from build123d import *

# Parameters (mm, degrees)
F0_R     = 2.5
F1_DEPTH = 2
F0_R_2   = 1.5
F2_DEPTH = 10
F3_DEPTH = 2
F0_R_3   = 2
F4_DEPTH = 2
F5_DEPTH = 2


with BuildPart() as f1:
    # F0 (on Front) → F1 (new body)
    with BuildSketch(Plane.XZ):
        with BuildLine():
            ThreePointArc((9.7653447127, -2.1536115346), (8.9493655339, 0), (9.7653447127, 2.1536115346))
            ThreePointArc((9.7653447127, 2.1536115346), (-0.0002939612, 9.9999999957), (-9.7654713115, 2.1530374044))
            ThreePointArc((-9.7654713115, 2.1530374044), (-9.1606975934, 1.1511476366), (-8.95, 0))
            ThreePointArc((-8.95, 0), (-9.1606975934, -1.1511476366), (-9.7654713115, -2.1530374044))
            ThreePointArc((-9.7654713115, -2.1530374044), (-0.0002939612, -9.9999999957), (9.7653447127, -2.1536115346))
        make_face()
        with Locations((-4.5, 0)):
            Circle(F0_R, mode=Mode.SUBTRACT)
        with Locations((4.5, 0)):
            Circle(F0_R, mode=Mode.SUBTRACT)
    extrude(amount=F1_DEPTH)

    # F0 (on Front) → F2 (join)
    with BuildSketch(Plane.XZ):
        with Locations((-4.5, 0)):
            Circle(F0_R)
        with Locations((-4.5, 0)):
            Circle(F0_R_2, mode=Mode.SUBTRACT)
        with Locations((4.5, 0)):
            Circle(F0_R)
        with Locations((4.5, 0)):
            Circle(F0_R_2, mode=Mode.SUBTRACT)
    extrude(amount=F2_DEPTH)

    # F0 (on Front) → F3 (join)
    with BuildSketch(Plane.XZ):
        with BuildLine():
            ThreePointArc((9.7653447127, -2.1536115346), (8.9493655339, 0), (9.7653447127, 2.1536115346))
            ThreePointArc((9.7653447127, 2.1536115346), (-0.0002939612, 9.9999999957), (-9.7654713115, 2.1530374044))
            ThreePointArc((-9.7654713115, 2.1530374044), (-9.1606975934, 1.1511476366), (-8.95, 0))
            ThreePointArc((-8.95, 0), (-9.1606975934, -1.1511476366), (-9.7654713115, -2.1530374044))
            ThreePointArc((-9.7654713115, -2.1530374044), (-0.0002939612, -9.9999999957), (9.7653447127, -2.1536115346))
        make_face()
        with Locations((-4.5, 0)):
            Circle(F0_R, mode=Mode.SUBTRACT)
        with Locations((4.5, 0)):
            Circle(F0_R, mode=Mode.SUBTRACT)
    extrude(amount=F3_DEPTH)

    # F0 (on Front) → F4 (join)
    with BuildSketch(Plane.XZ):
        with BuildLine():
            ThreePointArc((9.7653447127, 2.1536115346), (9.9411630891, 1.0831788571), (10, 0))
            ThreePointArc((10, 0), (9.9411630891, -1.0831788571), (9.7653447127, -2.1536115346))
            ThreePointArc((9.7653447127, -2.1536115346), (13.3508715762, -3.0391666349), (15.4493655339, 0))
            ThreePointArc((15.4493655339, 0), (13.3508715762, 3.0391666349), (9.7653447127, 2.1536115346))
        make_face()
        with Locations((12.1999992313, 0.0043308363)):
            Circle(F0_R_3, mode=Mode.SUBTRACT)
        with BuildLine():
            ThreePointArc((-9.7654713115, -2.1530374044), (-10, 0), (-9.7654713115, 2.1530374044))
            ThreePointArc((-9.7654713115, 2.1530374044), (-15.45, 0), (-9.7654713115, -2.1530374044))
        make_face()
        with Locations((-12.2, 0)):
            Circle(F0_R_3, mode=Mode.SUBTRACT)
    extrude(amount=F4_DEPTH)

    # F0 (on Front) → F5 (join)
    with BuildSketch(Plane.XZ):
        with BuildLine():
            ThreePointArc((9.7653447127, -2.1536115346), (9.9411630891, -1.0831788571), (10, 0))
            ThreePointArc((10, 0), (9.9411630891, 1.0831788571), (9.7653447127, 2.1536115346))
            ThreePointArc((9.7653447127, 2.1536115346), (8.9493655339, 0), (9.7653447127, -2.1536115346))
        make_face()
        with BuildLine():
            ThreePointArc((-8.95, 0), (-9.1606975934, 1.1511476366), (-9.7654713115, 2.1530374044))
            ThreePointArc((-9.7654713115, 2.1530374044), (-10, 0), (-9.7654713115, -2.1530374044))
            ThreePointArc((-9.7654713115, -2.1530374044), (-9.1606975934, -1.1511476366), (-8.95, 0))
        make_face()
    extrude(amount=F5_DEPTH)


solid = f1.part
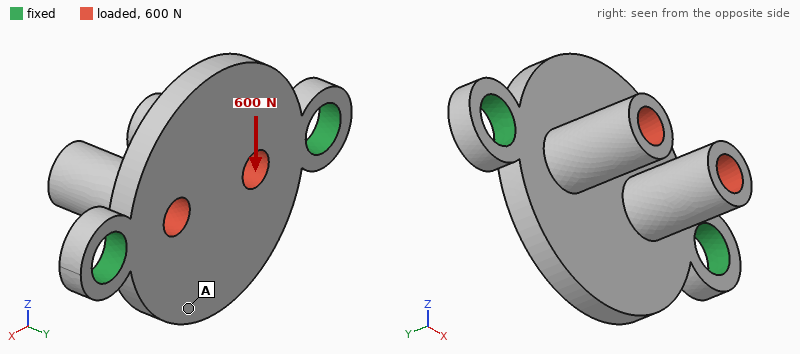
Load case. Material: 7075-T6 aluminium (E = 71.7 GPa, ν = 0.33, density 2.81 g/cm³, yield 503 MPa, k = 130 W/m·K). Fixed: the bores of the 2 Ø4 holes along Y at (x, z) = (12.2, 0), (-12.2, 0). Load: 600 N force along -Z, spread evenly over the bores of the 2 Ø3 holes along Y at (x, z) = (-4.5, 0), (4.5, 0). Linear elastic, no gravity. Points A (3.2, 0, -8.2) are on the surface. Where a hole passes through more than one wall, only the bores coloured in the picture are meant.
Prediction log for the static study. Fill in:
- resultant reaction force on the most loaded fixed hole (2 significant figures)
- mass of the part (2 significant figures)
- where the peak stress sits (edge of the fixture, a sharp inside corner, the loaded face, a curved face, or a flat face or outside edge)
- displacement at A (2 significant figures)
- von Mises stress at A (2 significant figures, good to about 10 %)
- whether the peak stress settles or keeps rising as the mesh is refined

300 N
2.4 g
a sharp inside corner
0.090 mm
40 MPa
keeps rising
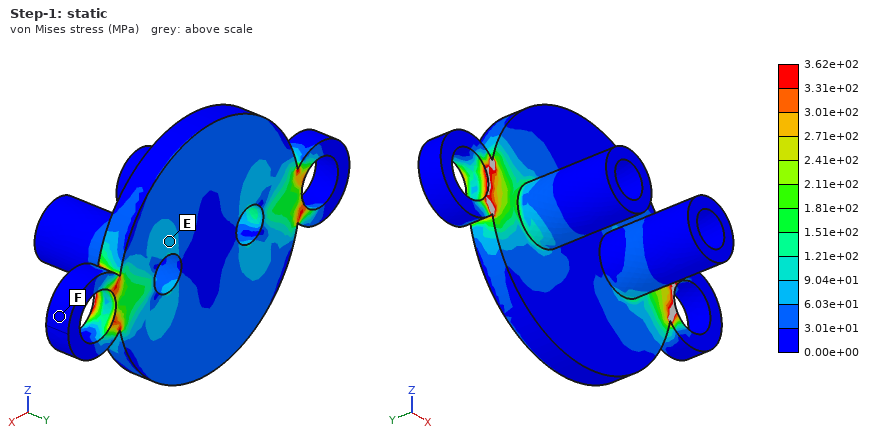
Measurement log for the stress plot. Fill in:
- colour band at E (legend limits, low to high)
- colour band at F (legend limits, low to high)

6.03e+01 to 9.04e+01 MPa
0.00e+00 to 3.01e+01 MPa
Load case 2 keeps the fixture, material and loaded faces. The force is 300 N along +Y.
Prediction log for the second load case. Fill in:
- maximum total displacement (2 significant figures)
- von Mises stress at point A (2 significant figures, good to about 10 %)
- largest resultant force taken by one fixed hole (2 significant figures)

31 µm
24 MPa
150 N
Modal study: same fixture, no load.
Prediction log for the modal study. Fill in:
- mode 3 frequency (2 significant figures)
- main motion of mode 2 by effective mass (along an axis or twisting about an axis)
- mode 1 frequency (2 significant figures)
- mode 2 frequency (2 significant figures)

24 kHz
along Y
9100 Hz
12 kHz
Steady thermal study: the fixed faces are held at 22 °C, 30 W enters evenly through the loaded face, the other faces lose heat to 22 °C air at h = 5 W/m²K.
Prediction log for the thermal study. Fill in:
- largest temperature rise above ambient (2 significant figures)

77 K
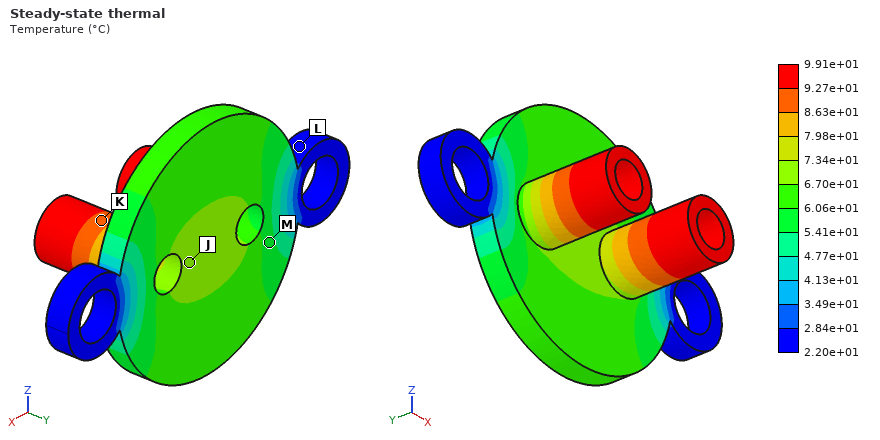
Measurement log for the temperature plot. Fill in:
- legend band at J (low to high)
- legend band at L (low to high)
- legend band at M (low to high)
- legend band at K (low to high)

6.70e+01 to 7.34e+01 °C
2.20e+01 to 2.84e+01 °C
5.41e+01 to 6.06e+01 °C
8.63e+01 to 9.27e+01 °C
